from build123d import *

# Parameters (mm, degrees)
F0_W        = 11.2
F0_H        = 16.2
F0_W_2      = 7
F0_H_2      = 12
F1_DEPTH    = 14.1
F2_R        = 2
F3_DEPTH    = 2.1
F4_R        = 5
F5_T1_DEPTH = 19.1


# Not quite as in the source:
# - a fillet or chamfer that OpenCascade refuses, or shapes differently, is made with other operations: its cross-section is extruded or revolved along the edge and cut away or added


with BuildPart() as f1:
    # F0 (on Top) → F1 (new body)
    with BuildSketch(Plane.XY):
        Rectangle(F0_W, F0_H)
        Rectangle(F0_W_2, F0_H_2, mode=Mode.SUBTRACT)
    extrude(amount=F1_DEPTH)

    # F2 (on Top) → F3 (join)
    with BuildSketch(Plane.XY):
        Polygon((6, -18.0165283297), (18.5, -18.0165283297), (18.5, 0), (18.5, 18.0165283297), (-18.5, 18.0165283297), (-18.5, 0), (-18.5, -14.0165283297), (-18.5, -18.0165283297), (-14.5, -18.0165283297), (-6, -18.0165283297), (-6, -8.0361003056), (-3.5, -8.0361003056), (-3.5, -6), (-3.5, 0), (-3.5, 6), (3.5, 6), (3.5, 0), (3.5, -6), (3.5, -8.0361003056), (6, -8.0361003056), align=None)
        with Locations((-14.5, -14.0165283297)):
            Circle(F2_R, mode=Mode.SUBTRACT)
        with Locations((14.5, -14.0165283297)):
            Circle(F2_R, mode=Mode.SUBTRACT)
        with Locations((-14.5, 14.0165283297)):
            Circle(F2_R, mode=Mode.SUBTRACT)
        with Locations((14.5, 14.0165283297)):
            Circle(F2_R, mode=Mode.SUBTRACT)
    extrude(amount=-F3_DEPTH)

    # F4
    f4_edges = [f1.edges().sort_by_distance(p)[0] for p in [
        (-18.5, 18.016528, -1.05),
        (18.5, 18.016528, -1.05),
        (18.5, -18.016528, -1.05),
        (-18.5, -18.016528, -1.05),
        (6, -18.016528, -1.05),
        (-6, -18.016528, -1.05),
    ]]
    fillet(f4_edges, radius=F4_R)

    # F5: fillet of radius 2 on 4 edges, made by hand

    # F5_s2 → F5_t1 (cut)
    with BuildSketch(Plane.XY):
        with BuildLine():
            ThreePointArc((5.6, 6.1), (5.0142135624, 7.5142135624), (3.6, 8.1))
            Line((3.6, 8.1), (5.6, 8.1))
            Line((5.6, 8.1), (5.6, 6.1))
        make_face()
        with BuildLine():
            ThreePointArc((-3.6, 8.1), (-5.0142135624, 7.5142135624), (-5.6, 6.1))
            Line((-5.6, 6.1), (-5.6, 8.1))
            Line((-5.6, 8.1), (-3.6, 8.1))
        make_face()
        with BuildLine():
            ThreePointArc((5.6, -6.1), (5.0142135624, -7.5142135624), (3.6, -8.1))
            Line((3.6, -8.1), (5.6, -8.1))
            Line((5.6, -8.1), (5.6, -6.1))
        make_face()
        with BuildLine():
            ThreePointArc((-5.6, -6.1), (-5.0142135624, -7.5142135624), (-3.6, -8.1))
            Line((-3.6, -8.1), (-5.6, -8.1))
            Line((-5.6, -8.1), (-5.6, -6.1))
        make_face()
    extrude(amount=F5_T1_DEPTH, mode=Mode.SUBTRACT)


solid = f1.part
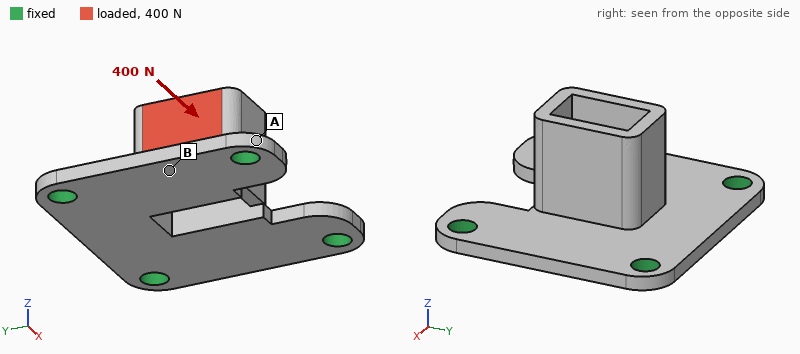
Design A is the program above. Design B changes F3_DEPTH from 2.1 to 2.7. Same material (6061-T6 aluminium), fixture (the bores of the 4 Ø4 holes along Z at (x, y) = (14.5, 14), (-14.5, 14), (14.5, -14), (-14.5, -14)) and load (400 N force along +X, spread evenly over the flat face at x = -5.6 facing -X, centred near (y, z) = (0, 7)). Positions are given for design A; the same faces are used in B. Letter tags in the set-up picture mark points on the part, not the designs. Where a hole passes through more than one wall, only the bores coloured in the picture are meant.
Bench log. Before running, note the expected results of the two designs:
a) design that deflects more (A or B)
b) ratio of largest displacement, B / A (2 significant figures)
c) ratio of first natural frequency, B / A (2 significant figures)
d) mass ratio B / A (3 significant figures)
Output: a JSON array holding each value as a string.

["A", "0.72", "1.3", "1.18"]
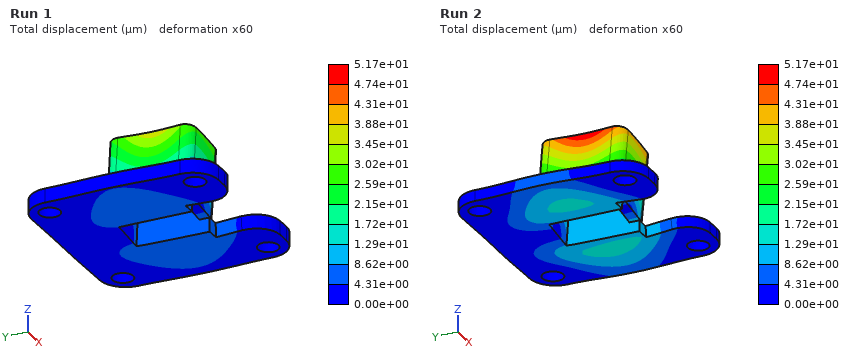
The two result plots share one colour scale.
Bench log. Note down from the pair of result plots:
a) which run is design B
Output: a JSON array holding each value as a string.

["Run 1"]
